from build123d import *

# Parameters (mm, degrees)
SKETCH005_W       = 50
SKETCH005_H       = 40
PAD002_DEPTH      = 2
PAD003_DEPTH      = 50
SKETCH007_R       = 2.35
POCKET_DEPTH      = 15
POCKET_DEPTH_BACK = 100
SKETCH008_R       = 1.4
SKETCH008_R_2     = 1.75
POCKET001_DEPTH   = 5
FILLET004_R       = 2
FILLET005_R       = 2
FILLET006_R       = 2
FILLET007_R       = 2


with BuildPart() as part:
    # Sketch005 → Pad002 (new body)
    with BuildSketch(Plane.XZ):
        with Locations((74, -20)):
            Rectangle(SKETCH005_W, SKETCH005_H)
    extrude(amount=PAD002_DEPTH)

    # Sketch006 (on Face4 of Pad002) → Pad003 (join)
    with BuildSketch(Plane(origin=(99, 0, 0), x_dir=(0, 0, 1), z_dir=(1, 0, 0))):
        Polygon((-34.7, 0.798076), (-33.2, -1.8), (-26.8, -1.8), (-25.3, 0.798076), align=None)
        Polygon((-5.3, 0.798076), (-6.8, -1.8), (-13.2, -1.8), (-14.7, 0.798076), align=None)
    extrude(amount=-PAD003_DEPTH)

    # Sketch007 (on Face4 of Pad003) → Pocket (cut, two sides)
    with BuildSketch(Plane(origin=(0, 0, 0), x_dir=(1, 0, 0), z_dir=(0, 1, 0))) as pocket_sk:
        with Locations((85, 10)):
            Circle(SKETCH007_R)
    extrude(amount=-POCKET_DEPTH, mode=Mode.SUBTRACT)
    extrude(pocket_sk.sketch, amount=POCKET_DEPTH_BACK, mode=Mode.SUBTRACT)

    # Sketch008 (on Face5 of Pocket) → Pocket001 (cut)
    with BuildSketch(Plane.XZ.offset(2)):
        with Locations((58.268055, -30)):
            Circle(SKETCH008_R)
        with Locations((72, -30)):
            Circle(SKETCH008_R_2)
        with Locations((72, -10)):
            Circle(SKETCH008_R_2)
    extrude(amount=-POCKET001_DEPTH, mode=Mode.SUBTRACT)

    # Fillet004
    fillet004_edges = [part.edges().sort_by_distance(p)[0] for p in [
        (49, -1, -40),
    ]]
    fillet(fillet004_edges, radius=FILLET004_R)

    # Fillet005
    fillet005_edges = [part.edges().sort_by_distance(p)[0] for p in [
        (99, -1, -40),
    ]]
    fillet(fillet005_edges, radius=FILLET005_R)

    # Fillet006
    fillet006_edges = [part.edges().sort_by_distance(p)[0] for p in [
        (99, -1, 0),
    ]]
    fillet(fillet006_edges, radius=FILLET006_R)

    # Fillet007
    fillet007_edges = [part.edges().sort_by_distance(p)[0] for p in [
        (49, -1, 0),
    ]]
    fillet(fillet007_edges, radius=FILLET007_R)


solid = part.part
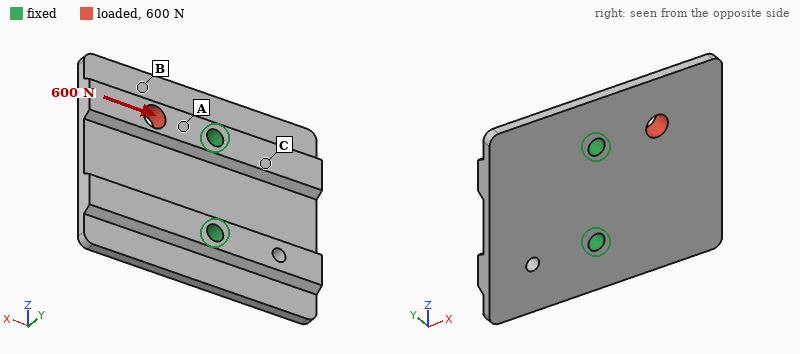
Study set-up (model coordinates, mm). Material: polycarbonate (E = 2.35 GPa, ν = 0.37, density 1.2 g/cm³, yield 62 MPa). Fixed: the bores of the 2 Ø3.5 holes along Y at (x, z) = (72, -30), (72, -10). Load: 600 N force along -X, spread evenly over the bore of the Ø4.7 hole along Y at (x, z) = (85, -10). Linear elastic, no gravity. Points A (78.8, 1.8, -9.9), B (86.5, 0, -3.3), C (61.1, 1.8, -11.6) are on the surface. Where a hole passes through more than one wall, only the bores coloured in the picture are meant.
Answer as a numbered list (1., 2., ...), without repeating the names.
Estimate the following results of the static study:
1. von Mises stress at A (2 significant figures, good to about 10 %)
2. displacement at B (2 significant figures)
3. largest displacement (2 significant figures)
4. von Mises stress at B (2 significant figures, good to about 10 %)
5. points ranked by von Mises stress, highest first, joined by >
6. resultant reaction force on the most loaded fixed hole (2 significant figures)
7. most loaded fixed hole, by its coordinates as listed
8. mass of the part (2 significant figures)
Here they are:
1. 20 MPa
2. 0.15 mm
3. 0.39 mm
4. 7.4 MPa
5. A > B > C
6. 580 N
7. (72, -10)
8. 6.2 g
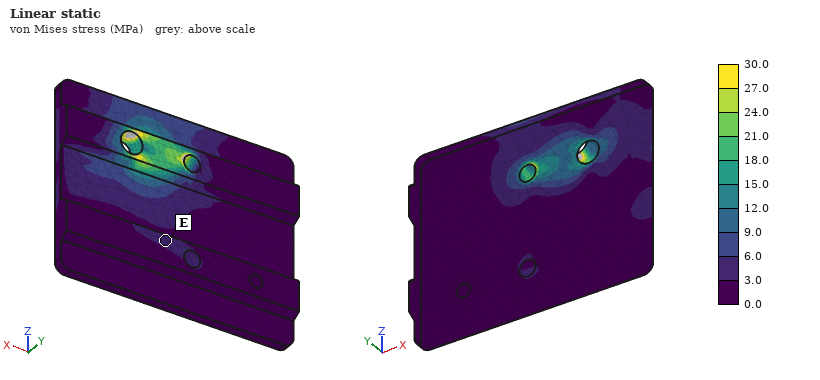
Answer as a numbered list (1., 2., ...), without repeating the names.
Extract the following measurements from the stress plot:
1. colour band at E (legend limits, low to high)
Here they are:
1. 3.0 to 6.0 MPa
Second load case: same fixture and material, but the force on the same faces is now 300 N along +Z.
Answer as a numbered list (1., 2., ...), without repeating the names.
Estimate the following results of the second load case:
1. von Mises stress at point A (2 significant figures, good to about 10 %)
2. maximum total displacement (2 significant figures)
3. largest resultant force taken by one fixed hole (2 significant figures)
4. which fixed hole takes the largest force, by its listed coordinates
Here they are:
1. 10 MPa
2. 0.24 mm
3. 240 N
4. (72, -10)
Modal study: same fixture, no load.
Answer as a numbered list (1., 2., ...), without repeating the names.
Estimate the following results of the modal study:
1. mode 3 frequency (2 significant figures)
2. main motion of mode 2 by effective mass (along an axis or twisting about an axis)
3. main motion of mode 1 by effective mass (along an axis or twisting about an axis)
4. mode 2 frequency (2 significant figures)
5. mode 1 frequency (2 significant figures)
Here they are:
1. 1600 Hz
2. along Y
3. along Y
4. 1500 Hz
5. 1100 Hz
